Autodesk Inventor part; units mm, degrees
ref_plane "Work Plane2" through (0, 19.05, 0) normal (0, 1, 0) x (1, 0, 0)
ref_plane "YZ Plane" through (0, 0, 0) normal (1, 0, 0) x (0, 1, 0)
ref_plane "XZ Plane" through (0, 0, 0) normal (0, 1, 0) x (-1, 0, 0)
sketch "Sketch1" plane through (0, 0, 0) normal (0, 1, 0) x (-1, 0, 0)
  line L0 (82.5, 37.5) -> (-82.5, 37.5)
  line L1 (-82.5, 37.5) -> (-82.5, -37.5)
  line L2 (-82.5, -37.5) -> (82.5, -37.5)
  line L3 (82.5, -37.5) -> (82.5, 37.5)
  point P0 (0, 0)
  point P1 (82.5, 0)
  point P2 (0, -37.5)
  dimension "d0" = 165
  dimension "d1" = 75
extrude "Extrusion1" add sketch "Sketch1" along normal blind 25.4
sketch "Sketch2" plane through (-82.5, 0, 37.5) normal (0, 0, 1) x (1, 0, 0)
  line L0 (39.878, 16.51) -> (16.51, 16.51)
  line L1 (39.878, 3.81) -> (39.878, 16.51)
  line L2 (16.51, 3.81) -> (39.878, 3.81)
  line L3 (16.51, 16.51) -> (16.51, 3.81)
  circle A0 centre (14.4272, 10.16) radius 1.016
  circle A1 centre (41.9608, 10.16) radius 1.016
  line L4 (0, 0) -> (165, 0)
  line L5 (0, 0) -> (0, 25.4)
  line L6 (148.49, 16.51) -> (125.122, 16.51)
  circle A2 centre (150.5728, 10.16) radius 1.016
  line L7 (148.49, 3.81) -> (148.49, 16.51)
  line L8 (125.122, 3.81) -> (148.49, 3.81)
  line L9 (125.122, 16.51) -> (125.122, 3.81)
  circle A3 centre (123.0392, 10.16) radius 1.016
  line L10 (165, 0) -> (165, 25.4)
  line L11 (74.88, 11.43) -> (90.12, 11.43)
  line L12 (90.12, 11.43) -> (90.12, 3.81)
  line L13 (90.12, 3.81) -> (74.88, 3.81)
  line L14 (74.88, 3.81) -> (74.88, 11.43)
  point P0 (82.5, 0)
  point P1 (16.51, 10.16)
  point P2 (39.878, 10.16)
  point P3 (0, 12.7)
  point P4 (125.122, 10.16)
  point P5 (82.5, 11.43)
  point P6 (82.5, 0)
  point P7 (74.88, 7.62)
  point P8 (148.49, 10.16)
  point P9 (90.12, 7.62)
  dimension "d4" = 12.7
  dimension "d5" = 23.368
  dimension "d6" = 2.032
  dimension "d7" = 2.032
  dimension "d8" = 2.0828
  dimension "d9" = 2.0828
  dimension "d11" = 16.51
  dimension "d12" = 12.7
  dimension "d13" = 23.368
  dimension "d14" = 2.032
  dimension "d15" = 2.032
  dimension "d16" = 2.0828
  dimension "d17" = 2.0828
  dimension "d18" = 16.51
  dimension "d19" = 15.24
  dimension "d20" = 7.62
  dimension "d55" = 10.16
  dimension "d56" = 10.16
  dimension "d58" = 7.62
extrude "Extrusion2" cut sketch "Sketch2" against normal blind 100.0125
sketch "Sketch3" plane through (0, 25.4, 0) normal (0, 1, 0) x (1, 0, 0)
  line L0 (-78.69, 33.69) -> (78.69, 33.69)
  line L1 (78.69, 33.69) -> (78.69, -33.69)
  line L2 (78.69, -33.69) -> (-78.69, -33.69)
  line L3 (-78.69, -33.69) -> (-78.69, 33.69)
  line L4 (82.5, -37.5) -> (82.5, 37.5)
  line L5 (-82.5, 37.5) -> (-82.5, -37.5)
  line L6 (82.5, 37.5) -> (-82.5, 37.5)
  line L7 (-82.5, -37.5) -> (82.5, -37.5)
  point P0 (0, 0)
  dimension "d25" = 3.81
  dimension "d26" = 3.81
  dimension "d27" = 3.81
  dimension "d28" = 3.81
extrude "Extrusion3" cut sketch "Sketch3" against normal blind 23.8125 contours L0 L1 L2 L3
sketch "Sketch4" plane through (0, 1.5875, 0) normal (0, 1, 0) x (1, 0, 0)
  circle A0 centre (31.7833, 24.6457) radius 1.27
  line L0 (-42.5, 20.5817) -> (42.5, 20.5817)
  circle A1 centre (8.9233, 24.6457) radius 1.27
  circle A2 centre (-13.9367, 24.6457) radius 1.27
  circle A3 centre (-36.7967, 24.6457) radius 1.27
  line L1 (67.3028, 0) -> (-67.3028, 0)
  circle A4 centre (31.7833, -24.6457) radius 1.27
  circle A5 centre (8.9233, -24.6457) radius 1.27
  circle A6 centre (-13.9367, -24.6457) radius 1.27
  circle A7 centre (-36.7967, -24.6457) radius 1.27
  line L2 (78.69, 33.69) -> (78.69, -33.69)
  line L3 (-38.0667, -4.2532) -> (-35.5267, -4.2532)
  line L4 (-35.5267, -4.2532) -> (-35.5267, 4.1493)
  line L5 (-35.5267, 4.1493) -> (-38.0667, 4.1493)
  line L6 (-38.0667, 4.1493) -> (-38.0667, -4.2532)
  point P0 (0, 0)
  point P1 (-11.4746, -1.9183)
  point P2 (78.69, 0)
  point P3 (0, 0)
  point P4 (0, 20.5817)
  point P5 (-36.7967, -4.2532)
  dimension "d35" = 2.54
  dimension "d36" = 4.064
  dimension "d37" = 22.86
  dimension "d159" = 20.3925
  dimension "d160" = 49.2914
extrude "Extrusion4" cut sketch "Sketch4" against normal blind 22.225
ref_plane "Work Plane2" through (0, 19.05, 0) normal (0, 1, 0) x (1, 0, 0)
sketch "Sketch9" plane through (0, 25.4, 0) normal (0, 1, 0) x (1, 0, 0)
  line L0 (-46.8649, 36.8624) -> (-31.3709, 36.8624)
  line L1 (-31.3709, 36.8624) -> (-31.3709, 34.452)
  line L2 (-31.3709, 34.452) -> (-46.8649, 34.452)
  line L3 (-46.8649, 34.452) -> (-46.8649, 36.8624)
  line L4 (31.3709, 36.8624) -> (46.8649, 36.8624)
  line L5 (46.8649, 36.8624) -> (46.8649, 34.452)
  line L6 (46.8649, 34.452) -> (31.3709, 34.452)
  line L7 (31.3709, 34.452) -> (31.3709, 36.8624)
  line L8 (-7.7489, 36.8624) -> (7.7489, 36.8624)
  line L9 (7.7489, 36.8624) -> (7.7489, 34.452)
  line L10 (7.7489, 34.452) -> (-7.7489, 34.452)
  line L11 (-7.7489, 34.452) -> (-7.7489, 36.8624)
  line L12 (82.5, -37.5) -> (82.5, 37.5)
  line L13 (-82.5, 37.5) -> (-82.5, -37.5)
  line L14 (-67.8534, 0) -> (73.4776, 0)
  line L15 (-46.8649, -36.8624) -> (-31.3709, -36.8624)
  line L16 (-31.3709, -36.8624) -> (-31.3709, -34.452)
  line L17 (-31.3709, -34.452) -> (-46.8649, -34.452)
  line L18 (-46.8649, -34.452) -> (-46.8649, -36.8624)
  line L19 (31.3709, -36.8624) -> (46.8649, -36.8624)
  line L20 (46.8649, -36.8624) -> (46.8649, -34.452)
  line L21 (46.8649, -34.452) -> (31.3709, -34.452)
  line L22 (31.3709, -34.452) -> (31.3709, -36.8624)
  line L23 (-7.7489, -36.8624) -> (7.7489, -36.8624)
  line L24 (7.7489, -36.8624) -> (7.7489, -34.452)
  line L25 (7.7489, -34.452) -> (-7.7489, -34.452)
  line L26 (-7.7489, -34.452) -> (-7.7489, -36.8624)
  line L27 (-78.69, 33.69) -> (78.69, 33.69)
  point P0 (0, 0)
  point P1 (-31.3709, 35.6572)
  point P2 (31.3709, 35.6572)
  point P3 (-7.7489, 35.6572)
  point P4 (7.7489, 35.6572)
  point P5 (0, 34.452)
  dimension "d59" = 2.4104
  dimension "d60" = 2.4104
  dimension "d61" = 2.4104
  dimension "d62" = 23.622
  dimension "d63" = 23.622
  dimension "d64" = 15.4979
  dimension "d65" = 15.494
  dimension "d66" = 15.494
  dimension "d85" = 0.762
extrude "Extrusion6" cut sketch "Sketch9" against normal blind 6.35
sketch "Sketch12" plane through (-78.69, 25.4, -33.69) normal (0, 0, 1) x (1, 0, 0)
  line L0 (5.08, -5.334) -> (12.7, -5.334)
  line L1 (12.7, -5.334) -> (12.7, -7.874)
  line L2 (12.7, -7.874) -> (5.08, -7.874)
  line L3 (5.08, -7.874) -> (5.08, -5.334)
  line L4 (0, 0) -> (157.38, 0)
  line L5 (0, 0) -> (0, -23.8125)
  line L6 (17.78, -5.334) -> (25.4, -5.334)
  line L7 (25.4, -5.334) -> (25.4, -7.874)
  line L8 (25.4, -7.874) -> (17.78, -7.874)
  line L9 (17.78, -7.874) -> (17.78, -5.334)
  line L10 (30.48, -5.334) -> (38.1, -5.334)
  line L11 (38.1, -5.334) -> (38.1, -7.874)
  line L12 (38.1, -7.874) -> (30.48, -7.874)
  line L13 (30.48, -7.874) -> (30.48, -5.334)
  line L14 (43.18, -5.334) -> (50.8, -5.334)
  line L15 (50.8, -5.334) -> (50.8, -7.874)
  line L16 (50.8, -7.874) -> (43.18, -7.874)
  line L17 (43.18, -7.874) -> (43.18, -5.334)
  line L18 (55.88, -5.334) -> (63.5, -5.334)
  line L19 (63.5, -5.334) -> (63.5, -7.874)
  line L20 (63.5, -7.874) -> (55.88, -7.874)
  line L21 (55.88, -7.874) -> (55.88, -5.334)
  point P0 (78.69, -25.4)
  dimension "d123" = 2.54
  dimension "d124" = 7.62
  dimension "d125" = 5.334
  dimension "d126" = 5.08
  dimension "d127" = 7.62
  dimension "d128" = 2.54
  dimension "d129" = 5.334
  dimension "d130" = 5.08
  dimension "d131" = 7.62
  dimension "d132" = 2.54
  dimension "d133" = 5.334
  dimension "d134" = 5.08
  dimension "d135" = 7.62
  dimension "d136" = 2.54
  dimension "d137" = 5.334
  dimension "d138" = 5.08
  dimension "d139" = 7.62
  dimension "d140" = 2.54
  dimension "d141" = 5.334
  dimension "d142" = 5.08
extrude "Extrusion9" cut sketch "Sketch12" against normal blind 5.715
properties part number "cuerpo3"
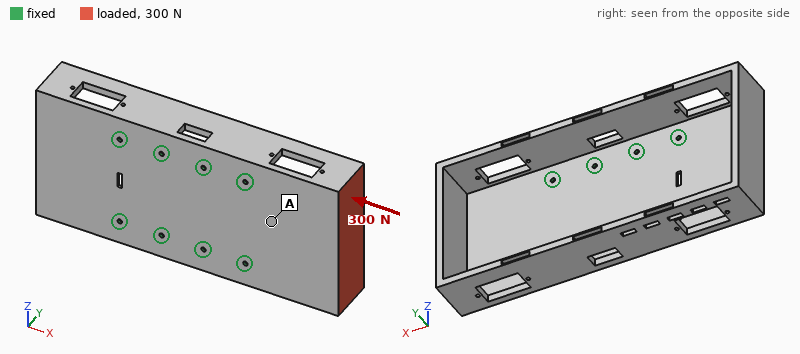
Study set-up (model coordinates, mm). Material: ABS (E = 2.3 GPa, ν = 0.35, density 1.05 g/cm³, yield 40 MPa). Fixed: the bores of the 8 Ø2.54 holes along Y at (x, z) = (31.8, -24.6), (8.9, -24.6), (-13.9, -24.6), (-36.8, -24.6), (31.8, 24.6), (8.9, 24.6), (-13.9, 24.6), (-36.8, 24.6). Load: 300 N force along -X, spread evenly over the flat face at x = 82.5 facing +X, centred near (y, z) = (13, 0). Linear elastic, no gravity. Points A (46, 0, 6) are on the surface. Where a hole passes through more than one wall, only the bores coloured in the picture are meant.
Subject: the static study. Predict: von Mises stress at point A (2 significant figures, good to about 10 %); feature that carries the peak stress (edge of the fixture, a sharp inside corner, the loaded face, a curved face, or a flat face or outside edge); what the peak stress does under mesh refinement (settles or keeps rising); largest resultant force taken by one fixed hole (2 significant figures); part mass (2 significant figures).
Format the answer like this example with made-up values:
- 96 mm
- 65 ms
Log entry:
- 2.1 MPa
- edge of the fixture
- keeps rising
- 62 N
- 57 g
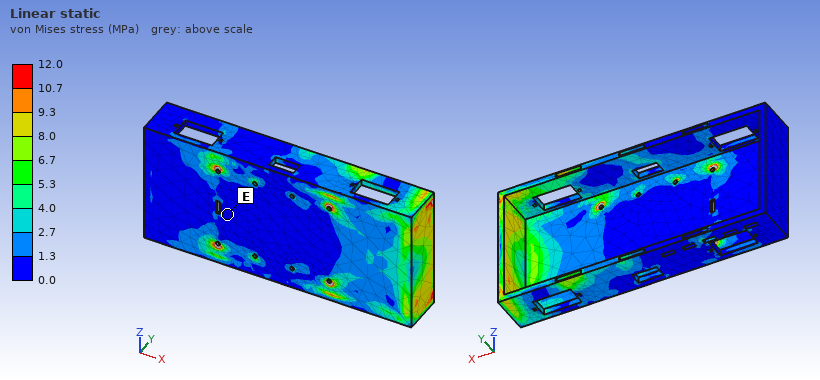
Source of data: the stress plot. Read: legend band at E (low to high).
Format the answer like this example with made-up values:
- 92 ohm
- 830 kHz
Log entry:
- 0.0 to 1.3 MPa
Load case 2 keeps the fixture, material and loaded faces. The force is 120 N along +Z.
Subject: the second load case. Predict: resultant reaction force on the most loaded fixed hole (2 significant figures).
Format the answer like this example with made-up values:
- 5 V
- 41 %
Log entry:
- 120 N
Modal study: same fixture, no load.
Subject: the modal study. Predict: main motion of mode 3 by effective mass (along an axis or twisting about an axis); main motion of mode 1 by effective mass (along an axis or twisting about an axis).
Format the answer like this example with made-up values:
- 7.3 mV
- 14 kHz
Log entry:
- along Z
- twisting about Z
